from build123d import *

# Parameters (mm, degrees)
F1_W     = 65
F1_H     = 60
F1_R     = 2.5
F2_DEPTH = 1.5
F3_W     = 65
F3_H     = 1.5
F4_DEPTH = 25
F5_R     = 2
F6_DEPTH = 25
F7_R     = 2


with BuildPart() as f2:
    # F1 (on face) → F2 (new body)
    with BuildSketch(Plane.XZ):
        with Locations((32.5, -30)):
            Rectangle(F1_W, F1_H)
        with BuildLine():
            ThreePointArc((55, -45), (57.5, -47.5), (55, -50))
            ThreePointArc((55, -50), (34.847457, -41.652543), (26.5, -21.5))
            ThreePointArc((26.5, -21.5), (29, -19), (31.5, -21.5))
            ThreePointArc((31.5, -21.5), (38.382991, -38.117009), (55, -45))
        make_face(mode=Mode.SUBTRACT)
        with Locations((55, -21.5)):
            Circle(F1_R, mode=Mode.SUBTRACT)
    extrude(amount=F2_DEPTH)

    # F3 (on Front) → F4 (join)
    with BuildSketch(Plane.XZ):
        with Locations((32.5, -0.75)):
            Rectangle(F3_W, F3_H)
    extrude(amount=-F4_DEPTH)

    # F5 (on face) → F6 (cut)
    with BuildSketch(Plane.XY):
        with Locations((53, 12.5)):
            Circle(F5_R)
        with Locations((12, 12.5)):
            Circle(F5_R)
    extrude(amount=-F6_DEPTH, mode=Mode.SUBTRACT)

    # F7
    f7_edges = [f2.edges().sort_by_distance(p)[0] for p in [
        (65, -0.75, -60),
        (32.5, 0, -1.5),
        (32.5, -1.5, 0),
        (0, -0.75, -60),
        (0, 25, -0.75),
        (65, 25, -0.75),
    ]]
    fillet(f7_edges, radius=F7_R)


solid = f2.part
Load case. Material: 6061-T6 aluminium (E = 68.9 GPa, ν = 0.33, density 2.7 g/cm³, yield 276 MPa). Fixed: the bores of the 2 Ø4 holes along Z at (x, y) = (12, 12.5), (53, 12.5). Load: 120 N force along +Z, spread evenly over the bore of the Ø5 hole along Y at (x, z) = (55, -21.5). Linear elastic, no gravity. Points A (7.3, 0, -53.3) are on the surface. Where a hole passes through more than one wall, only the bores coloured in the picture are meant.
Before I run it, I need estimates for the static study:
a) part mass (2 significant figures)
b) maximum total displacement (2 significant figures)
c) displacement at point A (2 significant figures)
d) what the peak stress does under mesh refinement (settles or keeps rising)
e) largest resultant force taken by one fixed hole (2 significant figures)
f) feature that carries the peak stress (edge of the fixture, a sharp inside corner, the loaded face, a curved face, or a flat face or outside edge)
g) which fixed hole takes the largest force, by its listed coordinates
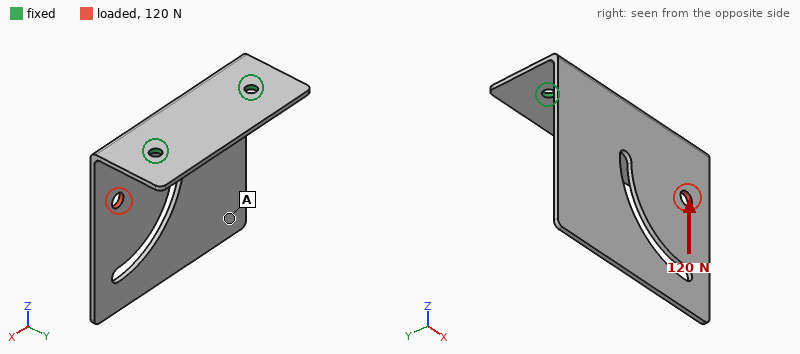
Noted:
21 g
0.67 mm
0.37 mm
keeps rising
120 N
edge of the fixture
(53, 12.5)
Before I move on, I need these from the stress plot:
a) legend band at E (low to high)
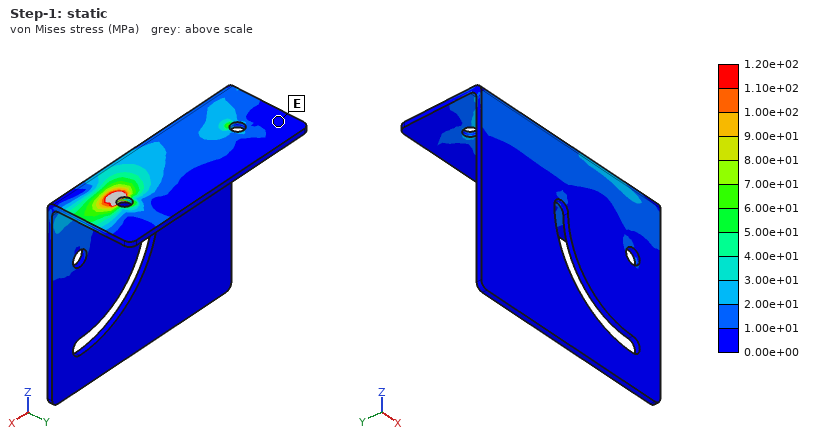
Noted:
0.00e+00 to 1.00e+01 MPa
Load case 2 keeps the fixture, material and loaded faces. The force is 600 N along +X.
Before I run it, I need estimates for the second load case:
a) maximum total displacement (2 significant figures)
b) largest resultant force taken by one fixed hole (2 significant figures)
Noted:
1.1 mm
450 N
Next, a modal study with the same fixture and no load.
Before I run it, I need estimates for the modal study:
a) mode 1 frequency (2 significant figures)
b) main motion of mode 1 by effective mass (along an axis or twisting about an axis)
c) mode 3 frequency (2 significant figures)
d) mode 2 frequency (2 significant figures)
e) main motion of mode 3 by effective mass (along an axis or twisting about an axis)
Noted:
270 Hz
along Y
1200 Hz
640 Hz
along X
